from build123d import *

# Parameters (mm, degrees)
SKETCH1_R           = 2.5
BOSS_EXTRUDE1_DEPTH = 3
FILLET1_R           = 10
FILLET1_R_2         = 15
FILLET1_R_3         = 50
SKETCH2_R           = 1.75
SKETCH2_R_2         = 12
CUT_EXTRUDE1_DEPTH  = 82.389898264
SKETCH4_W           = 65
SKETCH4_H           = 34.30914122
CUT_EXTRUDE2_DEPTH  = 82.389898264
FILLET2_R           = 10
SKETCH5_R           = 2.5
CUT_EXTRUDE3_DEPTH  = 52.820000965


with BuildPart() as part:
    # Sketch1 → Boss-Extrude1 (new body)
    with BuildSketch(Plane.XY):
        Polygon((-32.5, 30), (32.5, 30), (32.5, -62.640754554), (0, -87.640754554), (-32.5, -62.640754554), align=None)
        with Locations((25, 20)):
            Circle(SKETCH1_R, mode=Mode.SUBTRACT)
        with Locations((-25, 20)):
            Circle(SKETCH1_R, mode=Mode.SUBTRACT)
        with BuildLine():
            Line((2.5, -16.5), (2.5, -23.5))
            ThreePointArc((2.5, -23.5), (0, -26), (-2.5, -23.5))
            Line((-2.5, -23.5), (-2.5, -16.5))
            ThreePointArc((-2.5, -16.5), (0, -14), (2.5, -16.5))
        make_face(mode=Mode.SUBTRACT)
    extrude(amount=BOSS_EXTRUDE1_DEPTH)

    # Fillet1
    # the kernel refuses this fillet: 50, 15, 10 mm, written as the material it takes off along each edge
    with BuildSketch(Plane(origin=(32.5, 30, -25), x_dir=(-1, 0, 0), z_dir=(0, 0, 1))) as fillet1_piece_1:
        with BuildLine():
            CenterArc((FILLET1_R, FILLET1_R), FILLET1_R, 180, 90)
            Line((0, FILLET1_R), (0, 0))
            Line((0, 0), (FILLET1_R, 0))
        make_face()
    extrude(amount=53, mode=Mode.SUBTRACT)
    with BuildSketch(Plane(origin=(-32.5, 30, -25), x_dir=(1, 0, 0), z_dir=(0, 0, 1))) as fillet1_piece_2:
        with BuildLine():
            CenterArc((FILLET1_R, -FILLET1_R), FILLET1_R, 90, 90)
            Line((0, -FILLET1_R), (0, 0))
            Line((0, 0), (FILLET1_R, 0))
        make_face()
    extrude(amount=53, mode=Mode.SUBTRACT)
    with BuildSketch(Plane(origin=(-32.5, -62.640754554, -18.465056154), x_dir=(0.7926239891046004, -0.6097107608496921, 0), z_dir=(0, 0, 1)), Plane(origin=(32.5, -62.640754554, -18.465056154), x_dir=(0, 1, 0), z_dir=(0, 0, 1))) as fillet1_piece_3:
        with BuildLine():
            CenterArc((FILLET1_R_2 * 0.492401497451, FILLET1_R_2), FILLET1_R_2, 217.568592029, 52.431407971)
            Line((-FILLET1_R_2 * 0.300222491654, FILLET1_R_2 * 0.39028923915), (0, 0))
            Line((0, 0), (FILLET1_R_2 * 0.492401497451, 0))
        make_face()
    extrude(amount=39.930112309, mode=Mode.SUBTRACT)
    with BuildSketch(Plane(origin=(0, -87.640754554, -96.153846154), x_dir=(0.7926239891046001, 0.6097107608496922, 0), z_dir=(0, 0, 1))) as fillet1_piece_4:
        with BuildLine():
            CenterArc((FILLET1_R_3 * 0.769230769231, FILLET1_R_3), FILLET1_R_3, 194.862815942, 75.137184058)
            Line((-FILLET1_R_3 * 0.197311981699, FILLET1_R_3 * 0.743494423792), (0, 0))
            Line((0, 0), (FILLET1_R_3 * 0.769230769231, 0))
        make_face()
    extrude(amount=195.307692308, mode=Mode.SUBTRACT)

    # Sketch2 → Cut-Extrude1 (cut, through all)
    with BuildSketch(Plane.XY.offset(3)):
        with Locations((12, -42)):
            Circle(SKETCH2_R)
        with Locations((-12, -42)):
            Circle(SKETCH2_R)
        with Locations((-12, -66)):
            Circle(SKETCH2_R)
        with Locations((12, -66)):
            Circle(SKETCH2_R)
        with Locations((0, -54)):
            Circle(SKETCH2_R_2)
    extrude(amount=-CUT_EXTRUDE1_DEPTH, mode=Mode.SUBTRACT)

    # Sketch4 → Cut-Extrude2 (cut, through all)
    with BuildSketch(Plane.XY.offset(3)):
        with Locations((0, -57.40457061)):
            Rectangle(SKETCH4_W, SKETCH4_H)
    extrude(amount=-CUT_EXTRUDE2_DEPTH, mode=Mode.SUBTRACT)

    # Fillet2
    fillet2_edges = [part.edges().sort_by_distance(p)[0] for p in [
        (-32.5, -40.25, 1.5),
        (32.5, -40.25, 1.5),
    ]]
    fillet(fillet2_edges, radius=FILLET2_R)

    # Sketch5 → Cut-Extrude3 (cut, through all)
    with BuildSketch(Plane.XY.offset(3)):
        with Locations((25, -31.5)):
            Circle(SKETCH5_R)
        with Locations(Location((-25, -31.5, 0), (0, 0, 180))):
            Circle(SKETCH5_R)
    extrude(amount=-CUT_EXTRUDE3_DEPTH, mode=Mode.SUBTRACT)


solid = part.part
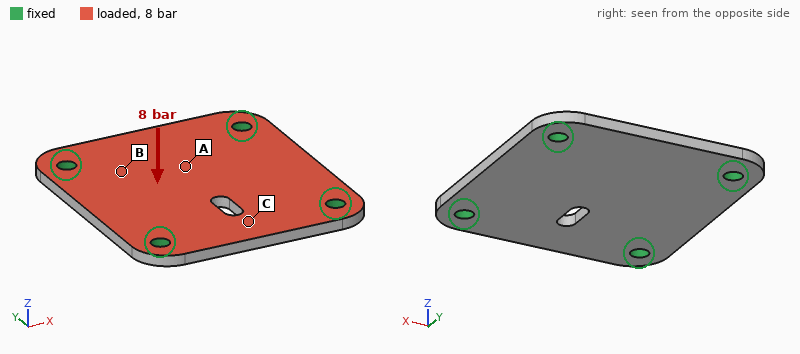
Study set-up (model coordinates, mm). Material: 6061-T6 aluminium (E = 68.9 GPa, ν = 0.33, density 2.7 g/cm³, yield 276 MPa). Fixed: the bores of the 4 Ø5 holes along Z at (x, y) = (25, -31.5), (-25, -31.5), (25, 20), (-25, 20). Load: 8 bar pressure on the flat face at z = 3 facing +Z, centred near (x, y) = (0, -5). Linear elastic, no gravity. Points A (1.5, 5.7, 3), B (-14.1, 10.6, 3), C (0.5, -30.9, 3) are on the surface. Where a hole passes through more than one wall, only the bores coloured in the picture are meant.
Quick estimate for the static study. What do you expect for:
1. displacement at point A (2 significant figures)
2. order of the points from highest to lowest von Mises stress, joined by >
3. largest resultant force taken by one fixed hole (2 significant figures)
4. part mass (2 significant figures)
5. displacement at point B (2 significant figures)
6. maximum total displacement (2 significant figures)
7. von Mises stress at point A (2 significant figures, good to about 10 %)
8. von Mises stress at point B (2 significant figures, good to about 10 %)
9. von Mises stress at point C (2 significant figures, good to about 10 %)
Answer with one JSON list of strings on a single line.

["0.16 mm", "C > A > B", "890 N", "35 g", "0.091 mm", "0.19 mm", "56 MPa", "22 MPa", "75 MPa"]
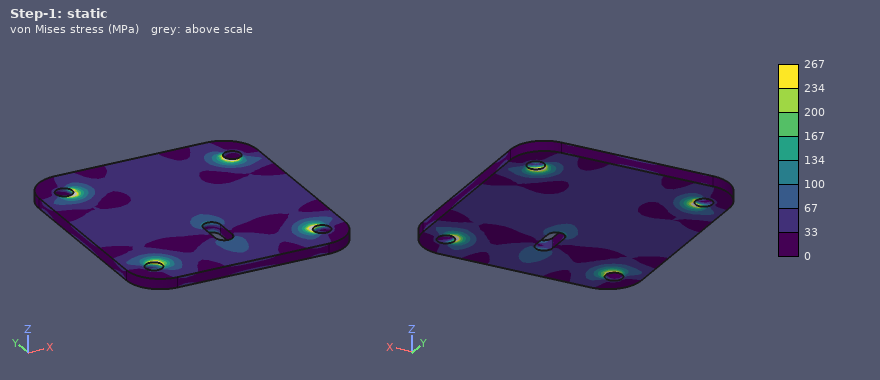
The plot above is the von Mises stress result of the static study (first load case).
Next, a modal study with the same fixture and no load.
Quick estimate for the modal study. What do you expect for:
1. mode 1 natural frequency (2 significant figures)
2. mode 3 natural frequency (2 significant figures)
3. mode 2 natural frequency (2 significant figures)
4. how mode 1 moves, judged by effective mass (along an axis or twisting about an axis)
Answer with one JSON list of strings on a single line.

["4500 Hz", "7000 Hz", "6900 Hz", "along Z"]
